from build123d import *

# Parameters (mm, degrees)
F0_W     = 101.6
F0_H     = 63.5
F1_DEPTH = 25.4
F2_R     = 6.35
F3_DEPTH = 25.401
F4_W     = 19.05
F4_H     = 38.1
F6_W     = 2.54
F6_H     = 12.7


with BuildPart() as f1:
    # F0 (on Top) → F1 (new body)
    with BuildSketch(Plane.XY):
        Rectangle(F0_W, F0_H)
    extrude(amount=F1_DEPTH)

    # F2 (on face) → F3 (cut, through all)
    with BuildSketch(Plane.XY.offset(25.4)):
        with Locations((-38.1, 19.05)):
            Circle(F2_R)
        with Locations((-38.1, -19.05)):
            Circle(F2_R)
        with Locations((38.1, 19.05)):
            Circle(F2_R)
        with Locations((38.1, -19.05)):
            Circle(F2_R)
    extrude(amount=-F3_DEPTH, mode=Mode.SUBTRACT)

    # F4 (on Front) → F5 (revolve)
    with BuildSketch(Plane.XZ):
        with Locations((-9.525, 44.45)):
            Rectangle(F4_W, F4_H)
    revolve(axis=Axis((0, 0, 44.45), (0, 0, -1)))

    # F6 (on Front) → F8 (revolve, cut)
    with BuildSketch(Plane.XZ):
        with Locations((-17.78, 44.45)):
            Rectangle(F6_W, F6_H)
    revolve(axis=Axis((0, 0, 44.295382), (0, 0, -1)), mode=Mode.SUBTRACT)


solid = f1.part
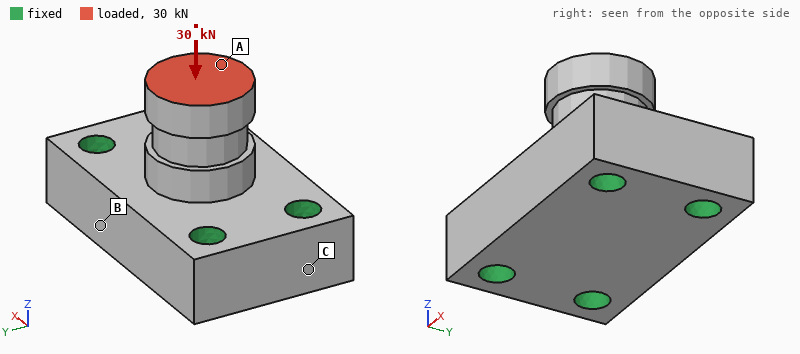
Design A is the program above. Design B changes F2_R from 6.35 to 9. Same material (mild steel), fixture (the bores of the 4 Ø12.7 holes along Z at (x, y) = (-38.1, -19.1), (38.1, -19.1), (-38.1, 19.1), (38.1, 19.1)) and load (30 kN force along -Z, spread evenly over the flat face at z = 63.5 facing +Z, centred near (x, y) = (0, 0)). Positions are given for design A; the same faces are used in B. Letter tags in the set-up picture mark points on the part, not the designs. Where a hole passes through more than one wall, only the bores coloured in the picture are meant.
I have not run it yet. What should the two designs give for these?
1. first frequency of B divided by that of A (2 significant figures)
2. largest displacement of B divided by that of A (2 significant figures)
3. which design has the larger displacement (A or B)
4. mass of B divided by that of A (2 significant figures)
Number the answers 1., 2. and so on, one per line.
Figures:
1. 1.0
2. 0.91
3. A
4. 0.93
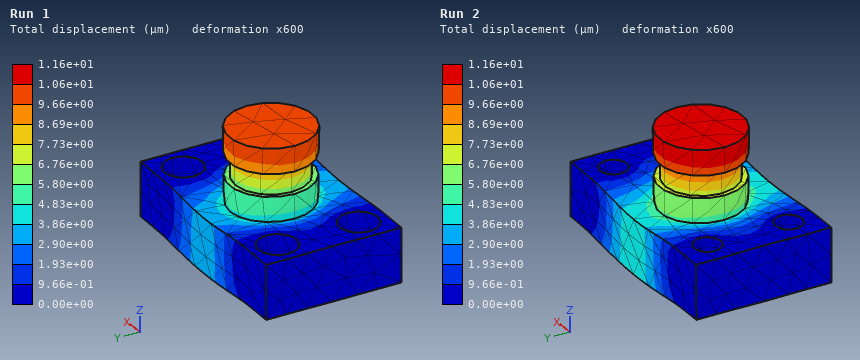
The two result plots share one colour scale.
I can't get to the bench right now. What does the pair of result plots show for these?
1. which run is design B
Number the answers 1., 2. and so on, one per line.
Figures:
1. Run 1
